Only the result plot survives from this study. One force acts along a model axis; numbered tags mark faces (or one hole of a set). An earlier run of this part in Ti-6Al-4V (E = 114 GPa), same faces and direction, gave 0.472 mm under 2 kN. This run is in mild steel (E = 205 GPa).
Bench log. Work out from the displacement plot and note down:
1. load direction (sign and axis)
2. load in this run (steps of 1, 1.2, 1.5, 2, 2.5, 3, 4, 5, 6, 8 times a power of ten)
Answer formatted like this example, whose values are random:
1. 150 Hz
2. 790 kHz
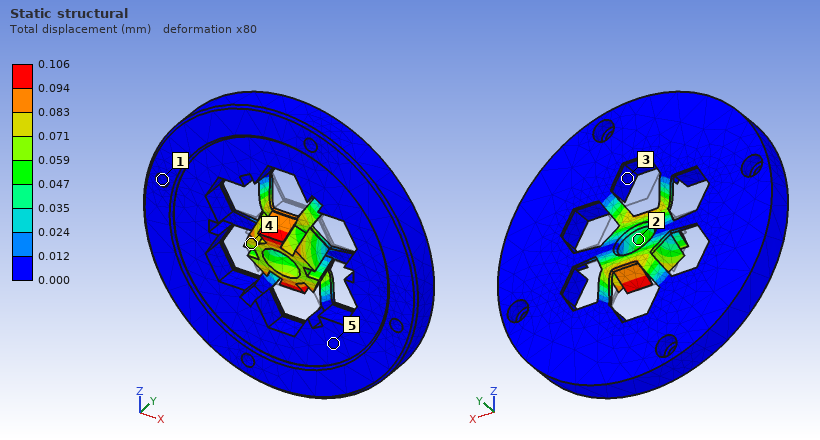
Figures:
1. -Z
2. 800 N
